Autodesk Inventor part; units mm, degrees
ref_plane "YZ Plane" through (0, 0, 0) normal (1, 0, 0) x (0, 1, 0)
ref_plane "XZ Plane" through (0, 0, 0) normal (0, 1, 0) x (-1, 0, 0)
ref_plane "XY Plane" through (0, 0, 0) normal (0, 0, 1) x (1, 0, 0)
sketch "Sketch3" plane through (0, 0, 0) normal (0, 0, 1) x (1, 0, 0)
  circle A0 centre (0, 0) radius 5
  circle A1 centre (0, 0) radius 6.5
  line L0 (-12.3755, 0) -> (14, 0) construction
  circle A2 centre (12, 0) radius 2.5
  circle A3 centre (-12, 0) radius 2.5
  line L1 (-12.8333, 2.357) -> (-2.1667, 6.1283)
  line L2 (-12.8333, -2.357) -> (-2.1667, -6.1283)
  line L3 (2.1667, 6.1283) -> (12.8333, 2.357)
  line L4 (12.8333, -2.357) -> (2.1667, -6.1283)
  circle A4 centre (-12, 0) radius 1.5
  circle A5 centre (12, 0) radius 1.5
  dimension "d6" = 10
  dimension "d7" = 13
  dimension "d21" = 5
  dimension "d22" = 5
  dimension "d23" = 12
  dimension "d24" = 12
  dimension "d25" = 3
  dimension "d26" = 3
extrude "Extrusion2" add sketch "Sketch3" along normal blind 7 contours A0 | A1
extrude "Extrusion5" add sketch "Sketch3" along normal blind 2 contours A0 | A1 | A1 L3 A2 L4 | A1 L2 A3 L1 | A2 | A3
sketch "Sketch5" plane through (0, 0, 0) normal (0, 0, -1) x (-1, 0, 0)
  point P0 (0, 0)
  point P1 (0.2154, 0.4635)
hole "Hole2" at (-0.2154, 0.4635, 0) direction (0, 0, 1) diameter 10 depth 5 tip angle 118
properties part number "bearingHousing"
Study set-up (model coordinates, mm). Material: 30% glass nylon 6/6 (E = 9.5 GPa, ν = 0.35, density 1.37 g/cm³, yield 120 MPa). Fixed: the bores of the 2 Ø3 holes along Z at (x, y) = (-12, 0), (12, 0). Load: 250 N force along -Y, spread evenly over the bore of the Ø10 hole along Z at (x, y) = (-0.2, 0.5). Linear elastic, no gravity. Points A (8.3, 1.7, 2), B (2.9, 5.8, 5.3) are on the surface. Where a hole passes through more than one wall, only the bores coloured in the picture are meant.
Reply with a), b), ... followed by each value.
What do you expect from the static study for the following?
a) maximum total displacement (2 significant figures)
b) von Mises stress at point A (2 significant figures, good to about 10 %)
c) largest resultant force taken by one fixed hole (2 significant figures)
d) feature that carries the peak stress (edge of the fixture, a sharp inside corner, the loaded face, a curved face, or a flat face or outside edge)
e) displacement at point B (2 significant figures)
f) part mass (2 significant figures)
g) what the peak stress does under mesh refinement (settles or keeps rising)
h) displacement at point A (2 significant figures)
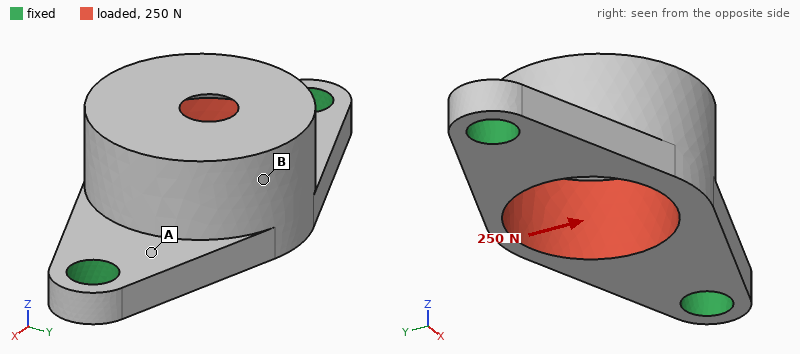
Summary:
a) 0.15 mm
b) 41 MPa
c) 130 N
d) edge of the fixture
e) 0.13 mm
f) 0.91 g
g) keeps rising
h) 0.026 mm
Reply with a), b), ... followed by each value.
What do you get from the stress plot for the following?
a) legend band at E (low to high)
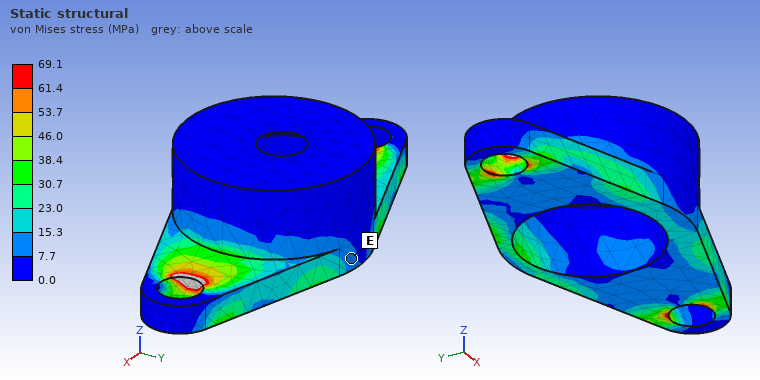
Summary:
a) 7.7 to 15.3 MPa
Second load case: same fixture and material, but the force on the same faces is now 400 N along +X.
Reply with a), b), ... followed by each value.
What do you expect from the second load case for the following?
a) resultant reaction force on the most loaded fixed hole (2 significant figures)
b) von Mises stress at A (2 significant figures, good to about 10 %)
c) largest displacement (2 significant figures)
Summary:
a) 210 N
b) 20 MPa
c) 26 µm
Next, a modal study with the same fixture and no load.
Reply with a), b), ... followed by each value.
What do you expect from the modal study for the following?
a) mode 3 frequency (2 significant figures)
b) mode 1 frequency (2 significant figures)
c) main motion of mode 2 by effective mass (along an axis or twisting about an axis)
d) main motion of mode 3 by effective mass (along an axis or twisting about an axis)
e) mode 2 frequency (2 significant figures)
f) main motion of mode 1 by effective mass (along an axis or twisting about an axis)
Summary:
a) 17 kHz
b) 5800 Hz
c) along Z
d) along X
e) 11 kHz
f) along Y
